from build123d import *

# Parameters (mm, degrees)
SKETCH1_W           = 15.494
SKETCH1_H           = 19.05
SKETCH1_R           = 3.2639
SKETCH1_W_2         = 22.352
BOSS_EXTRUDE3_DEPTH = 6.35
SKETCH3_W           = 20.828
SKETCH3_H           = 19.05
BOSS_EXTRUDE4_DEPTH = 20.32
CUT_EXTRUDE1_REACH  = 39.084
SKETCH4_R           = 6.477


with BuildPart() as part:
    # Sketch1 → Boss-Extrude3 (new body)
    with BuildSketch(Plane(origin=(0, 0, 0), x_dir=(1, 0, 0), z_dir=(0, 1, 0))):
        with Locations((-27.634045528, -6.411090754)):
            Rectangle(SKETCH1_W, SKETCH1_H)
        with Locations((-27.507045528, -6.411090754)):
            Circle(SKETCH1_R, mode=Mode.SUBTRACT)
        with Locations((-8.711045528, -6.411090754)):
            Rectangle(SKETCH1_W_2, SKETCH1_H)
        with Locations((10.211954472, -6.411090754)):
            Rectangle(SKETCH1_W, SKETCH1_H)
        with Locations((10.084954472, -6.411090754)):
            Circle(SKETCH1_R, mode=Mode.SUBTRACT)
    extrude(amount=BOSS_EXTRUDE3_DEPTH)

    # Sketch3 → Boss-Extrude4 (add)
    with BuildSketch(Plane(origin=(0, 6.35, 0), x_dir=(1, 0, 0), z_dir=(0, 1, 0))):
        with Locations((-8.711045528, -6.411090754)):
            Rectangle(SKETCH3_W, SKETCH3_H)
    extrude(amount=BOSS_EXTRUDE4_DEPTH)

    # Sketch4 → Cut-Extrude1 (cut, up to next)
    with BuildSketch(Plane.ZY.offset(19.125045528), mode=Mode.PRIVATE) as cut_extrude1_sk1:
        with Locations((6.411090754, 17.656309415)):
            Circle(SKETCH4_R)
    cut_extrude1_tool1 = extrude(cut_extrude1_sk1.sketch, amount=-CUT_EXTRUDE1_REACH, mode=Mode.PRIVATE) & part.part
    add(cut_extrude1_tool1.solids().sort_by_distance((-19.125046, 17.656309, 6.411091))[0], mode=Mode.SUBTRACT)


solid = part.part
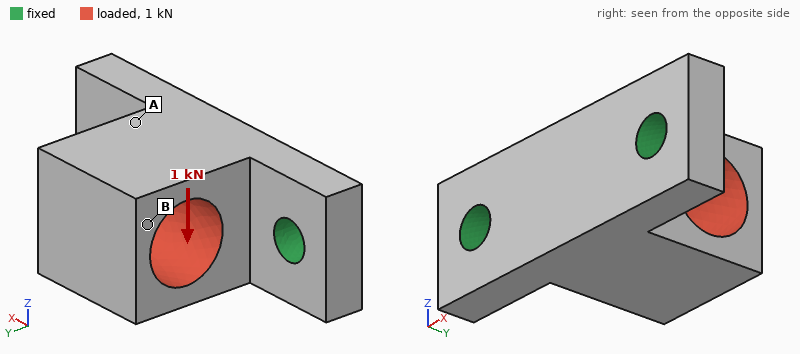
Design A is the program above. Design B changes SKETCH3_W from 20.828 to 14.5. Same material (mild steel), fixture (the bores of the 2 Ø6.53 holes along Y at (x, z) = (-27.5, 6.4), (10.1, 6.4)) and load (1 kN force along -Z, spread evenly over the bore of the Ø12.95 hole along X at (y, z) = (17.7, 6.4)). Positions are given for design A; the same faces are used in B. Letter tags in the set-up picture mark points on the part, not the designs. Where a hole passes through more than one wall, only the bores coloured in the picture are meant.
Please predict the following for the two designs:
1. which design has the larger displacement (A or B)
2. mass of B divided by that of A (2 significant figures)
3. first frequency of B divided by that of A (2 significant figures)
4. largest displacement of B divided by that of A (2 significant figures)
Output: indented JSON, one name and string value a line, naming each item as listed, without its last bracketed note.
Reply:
{
  "which design has the larger displacement": "B",
  "mass of B divided by that of A": "0.86",
  "first frequency of B divided by that of A": "1.0",
  "largest displacement of B divided by that of A": "1.4"
}
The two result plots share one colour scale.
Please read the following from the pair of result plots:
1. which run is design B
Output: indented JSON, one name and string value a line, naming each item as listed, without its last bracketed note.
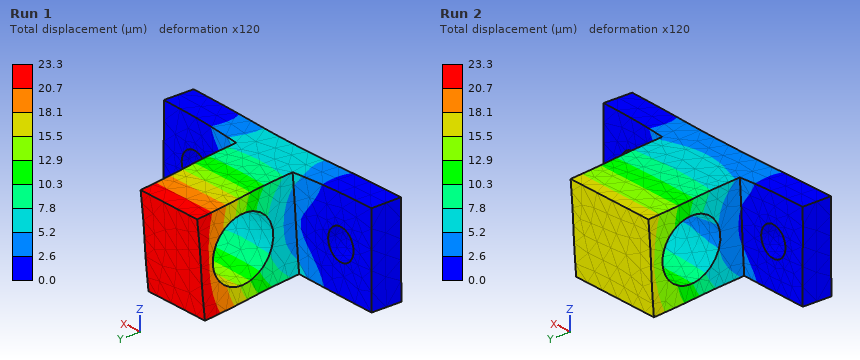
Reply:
{
  "which run is design B": "Run 1"
}
